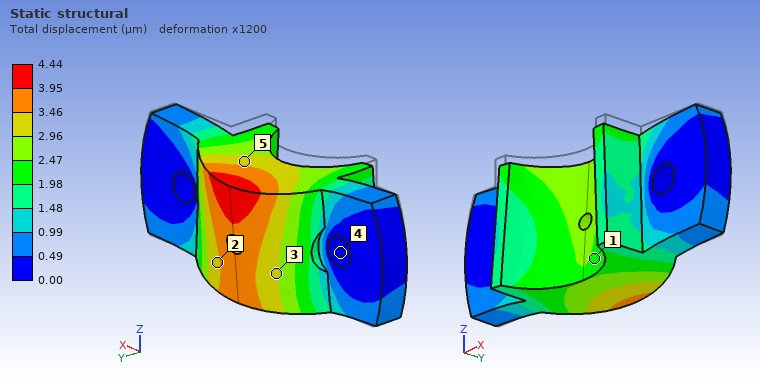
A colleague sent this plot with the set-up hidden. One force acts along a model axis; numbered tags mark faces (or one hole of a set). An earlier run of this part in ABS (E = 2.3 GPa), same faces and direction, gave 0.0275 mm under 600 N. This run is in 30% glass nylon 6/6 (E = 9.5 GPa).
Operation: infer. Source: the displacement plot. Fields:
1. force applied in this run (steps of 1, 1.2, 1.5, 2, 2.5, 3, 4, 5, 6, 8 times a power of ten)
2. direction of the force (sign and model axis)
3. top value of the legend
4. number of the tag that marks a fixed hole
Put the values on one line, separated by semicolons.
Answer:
400 N; -Z; 4.44 µm; 4
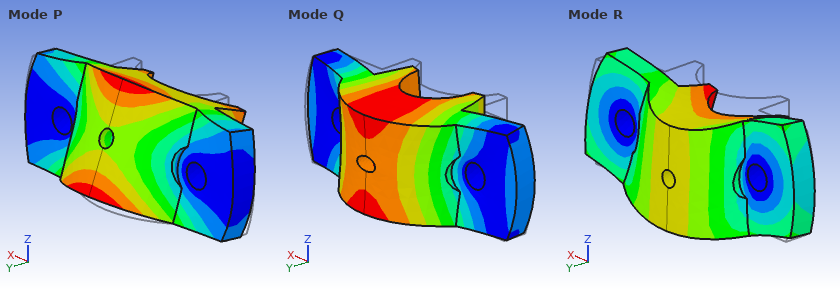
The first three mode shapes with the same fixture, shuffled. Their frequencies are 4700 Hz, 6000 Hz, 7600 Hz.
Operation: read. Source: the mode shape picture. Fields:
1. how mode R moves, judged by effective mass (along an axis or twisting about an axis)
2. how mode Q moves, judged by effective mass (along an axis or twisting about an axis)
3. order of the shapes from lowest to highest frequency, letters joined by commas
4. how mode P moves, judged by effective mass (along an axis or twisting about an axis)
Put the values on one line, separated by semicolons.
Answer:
along Z; along Y; P, Q, R; twisting about X
